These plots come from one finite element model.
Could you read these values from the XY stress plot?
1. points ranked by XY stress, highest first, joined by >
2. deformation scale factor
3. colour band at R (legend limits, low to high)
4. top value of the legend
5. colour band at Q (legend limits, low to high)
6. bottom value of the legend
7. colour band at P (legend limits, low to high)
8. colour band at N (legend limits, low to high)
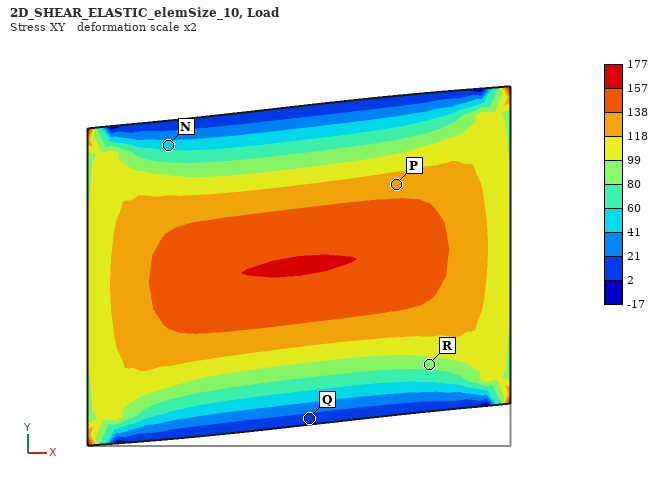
P > R > N > Q
2
80 to 99
177
2 to 21
-17
118 to 138
41 to 60
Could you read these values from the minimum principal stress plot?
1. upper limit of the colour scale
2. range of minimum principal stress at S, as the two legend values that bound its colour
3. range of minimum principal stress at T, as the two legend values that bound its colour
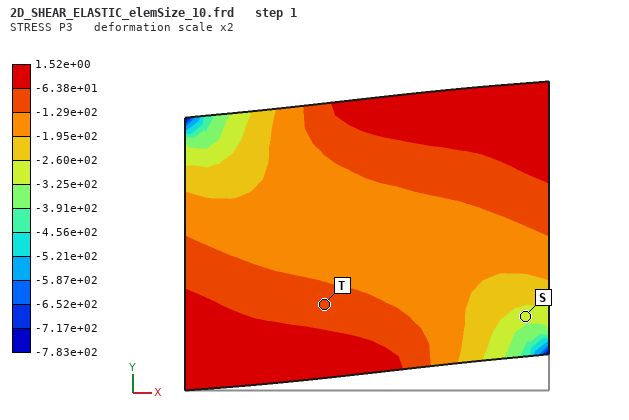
1.52e+00
-3.25e+02 to -2.60e+02
-1.29e+02 to -6.38e+01
